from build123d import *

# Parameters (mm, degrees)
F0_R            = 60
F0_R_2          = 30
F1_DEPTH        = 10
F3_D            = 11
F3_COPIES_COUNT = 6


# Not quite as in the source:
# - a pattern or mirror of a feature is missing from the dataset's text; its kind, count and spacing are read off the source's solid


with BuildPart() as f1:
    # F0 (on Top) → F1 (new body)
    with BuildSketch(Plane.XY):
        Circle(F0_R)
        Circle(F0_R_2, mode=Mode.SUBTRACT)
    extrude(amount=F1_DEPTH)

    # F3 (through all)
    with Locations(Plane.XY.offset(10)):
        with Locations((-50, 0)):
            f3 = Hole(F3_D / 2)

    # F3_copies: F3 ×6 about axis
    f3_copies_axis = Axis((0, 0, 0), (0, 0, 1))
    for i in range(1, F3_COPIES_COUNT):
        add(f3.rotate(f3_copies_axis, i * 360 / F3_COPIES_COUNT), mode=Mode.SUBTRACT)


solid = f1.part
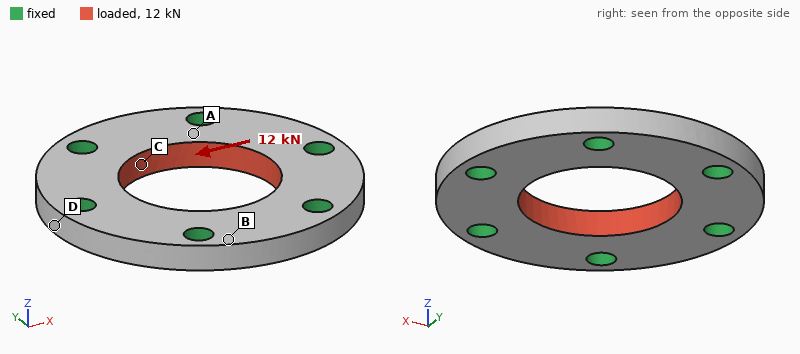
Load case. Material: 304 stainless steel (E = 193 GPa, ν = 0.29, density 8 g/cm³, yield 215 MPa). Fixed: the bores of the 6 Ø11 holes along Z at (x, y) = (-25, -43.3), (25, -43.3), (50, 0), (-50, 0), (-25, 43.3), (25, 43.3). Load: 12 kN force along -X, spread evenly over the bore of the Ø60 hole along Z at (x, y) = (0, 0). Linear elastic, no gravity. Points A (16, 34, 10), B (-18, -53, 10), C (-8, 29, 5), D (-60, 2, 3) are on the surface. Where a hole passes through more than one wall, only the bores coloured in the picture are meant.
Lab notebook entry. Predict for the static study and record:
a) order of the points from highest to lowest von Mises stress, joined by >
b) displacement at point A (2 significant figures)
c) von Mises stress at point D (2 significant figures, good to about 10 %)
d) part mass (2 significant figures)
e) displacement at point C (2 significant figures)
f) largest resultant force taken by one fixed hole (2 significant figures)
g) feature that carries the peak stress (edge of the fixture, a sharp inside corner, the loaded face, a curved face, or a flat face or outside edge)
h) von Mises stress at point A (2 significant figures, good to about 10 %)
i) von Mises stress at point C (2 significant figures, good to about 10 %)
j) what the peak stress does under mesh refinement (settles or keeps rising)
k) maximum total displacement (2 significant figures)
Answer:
C > A > D > B
0.50 µm
4.1 MPa
630 g
0.98 µm
2.6 kN
edge of the fixture
8.2 MPa
11 MPa
keeps rising
1.2 µm
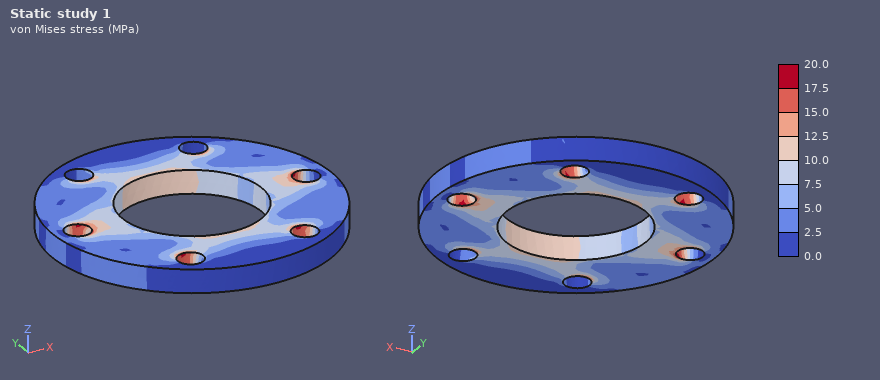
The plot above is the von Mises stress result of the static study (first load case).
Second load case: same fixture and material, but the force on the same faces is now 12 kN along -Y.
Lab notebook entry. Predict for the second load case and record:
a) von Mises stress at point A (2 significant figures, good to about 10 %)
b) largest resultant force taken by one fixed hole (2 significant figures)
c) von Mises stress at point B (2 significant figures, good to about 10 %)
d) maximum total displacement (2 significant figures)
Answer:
8.2 MPa
2.4 kN
4.4 MPa
1.3 µm
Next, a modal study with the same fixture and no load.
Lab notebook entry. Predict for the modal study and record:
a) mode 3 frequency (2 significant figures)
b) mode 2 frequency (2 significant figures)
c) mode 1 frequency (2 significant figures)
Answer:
18 kHz
18 kHz
18 kHz
